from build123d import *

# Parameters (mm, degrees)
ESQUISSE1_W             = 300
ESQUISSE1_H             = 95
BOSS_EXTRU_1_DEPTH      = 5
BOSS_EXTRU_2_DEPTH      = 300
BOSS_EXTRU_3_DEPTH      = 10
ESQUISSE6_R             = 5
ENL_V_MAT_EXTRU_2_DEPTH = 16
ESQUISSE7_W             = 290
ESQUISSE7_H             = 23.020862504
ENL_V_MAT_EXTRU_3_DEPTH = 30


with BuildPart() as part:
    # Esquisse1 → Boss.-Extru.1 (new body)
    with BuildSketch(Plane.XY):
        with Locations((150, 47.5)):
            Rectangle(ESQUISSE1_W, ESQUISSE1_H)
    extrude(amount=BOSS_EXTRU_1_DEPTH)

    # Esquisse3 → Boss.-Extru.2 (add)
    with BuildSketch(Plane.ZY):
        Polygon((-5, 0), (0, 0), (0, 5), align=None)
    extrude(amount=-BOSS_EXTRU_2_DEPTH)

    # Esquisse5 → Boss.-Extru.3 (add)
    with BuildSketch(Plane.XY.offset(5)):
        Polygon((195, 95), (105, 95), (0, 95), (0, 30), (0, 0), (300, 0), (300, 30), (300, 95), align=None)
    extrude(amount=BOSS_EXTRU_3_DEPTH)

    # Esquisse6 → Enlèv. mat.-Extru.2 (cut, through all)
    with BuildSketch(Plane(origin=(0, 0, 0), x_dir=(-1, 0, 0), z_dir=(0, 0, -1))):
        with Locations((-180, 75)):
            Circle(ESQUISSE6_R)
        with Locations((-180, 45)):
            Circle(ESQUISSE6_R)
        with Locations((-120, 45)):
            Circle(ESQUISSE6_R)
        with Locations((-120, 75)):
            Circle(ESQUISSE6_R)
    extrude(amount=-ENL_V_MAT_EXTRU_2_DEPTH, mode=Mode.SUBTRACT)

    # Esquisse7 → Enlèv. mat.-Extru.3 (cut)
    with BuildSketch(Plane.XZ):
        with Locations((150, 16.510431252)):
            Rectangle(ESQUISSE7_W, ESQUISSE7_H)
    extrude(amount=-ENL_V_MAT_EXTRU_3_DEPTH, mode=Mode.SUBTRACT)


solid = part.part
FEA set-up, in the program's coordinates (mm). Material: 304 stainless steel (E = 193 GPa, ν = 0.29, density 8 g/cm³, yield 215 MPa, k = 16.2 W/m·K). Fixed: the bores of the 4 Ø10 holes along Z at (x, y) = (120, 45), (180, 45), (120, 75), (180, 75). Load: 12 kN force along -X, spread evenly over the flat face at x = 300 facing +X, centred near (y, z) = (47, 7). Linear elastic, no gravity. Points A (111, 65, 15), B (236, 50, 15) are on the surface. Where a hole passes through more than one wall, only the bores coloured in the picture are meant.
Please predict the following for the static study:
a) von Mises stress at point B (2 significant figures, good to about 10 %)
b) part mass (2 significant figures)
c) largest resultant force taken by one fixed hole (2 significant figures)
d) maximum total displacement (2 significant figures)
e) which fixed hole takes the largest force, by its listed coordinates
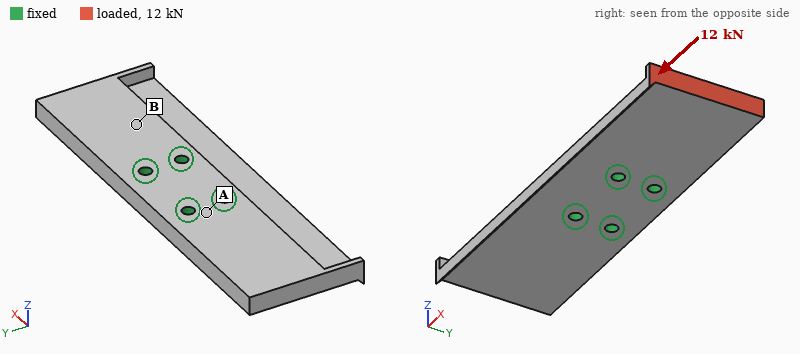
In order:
18 MPa
2.7 kg
7.6 kN
65 µm
(180, 45)
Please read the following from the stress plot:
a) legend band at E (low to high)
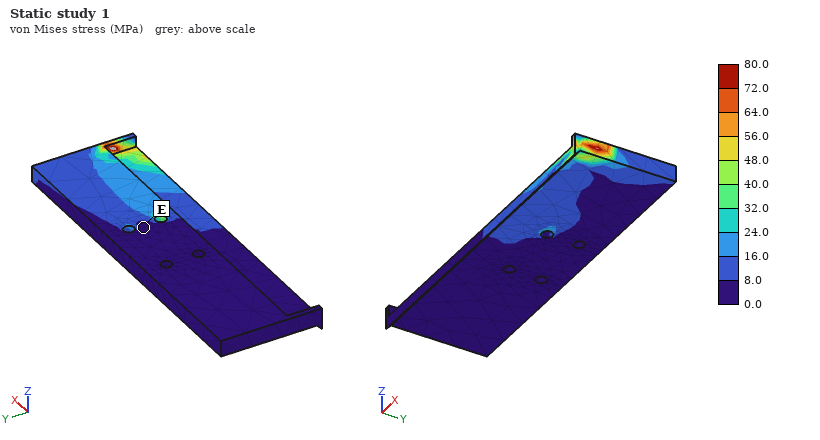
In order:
0.0 to 8.0 MPa
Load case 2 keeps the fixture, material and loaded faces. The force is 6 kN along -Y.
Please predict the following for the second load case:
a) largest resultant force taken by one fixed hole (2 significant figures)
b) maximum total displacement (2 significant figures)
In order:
13 kN
72 µm
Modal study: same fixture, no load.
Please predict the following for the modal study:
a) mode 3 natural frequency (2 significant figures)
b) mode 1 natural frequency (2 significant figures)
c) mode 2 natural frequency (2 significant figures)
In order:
2000 Hz
790 Hz
790 Hz
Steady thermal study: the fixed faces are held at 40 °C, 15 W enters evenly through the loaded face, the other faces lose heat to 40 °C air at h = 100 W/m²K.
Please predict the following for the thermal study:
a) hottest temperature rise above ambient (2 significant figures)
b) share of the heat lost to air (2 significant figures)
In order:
27 K
97 %
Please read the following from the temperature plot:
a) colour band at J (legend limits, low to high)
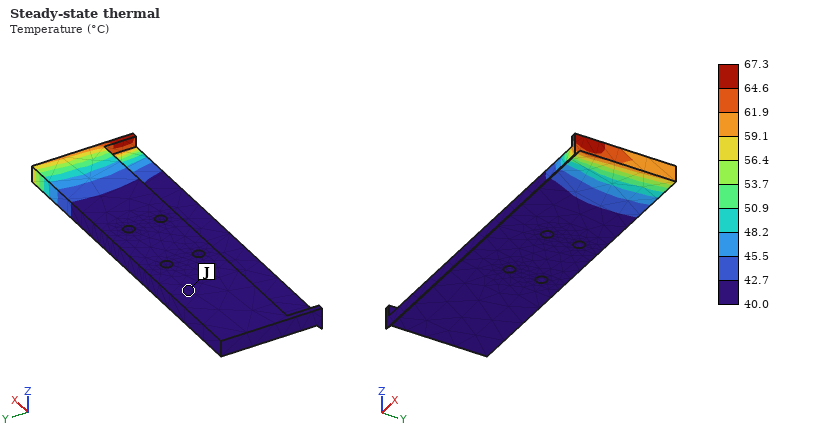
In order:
40.0 to 42.7 °C
